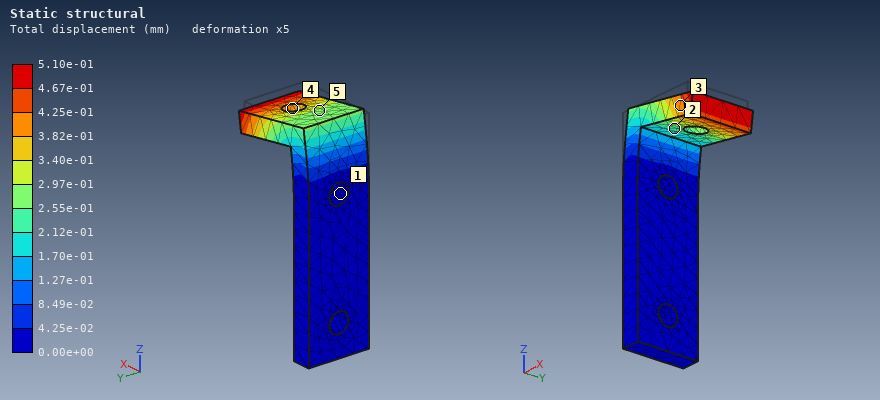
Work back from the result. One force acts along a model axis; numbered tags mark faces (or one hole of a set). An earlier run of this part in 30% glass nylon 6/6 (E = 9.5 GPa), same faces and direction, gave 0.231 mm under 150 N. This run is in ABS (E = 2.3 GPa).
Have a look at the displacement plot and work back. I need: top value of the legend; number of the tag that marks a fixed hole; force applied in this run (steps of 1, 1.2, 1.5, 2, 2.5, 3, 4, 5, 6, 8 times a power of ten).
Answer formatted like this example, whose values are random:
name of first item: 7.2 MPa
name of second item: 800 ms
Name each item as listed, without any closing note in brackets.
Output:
top value of the legend: 5.10e-01 mm
number of the tag that marks a fixed hole: 1
force applied in this run: 80 N
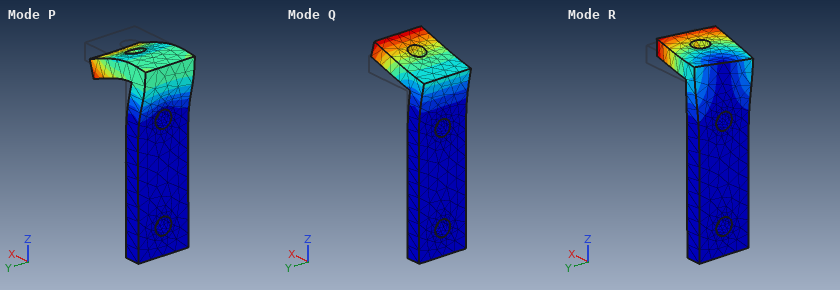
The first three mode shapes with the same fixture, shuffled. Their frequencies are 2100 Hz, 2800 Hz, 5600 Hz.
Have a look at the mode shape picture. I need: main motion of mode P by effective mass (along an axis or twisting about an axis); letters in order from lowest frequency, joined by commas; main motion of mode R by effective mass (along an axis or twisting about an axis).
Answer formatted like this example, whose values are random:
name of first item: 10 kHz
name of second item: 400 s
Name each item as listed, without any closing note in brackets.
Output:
main motion of mode P by effective mass: along X
letters in order from lowest frequency, joined by commas: Q, R, P
main motion of mode R by effective mass: along Y
